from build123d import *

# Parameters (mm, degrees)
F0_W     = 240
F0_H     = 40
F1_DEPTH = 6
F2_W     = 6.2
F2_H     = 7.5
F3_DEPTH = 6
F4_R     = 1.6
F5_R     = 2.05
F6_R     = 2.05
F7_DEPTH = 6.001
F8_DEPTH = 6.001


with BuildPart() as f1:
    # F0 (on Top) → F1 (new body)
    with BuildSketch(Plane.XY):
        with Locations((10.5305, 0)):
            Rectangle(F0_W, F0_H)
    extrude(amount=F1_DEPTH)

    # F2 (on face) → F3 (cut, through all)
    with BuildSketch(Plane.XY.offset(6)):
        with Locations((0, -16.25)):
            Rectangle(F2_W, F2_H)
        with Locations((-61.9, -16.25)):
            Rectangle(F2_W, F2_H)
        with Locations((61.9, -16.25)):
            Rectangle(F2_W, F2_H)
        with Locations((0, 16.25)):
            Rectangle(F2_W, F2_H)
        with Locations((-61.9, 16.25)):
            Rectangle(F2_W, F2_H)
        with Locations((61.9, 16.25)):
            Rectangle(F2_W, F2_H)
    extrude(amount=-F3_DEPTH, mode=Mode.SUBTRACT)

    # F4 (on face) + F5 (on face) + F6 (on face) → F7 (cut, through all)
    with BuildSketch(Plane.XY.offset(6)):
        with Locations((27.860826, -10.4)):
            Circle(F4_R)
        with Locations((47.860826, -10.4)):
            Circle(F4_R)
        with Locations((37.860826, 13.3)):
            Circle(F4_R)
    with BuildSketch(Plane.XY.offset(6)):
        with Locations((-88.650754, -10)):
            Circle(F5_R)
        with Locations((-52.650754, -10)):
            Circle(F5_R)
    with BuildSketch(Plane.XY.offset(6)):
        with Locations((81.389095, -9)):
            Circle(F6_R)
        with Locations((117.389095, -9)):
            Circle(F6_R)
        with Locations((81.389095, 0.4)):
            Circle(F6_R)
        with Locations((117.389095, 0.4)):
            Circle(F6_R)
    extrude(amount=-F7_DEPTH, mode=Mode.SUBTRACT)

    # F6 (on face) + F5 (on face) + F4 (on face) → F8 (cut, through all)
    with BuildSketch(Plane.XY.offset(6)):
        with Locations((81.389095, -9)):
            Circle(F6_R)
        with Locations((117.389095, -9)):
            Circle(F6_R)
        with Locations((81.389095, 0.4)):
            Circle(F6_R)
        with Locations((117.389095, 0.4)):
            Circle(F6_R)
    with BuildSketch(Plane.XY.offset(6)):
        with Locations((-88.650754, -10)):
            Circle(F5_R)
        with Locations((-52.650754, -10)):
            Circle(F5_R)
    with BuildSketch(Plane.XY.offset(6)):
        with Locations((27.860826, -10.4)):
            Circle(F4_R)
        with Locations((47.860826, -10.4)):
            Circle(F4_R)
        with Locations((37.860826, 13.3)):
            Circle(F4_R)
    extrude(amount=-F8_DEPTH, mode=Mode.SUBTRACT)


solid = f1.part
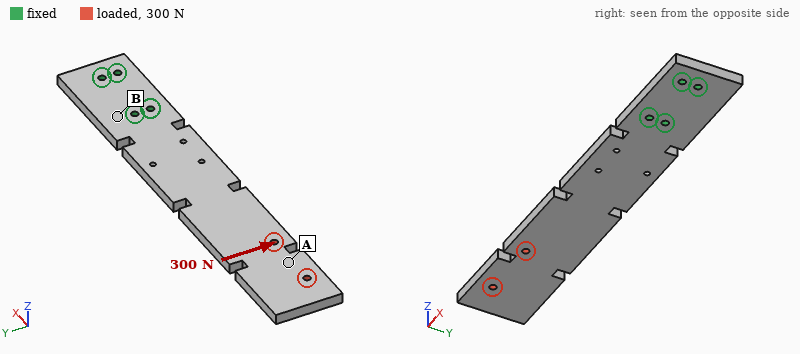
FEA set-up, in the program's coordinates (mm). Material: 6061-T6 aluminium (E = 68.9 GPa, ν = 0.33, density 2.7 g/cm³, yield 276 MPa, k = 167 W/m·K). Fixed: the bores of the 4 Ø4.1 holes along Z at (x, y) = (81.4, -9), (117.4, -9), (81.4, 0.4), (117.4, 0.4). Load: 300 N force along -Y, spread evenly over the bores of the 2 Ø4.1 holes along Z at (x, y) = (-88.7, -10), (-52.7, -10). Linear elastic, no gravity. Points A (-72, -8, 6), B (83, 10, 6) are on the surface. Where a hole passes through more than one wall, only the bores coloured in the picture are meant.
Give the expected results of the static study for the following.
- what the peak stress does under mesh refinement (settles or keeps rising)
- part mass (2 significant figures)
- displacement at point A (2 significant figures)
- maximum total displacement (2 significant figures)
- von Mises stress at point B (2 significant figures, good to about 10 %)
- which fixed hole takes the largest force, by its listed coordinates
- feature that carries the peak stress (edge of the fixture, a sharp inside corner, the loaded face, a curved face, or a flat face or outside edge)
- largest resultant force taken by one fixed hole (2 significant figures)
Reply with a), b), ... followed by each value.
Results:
a) keeps rising
b) 150 g
c) 0.39 mm
d) 0.52 mm
e) 16 MPa
f) (81.4, -9)
g) edge of the fixture
h) 1.8 kN
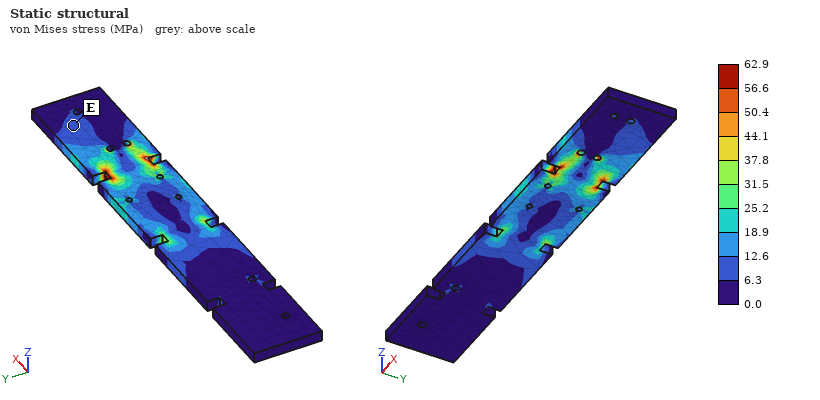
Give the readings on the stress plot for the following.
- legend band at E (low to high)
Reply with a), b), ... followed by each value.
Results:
a) 6.3 to 12.6 MPa
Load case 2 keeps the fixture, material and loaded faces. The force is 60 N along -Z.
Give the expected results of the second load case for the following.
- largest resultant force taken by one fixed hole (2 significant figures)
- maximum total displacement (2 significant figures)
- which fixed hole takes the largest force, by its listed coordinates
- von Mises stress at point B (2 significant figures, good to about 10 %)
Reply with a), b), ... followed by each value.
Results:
a) 71 N
b) 2.4 mm
c) (81.4, 0.4)
d) 15 MPa
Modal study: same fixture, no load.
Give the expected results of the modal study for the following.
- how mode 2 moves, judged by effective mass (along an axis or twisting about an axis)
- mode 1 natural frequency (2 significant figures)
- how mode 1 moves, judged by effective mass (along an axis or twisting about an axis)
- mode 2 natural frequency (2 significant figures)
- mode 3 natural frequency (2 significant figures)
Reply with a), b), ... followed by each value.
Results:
a) along Y
b) 120 Hz
c) along Z
d) 580 Hz
e) 780 Hz
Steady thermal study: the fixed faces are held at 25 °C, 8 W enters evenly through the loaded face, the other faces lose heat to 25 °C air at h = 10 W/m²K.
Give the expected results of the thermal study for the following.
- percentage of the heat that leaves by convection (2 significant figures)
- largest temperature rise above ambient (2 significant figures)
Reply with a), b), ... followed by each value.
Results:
a) 34 %
b) 27 K
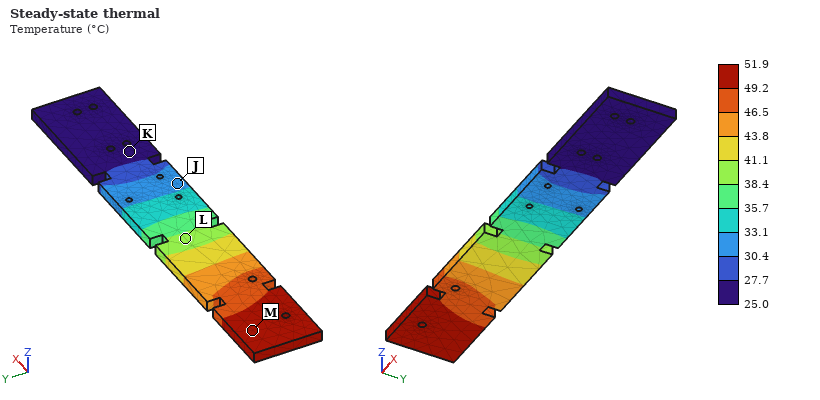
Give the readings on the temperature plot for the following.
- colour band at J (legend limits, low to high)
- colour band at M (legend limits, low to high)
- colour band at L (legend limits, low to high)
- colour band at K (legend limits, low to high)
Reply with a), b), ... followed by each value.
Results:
a) 30.4 to 33.1 °C
b) 49.2 to 51.9 °C
c) 38.4 to 41.1 °C
d) 25.0 to 27.7 °C
